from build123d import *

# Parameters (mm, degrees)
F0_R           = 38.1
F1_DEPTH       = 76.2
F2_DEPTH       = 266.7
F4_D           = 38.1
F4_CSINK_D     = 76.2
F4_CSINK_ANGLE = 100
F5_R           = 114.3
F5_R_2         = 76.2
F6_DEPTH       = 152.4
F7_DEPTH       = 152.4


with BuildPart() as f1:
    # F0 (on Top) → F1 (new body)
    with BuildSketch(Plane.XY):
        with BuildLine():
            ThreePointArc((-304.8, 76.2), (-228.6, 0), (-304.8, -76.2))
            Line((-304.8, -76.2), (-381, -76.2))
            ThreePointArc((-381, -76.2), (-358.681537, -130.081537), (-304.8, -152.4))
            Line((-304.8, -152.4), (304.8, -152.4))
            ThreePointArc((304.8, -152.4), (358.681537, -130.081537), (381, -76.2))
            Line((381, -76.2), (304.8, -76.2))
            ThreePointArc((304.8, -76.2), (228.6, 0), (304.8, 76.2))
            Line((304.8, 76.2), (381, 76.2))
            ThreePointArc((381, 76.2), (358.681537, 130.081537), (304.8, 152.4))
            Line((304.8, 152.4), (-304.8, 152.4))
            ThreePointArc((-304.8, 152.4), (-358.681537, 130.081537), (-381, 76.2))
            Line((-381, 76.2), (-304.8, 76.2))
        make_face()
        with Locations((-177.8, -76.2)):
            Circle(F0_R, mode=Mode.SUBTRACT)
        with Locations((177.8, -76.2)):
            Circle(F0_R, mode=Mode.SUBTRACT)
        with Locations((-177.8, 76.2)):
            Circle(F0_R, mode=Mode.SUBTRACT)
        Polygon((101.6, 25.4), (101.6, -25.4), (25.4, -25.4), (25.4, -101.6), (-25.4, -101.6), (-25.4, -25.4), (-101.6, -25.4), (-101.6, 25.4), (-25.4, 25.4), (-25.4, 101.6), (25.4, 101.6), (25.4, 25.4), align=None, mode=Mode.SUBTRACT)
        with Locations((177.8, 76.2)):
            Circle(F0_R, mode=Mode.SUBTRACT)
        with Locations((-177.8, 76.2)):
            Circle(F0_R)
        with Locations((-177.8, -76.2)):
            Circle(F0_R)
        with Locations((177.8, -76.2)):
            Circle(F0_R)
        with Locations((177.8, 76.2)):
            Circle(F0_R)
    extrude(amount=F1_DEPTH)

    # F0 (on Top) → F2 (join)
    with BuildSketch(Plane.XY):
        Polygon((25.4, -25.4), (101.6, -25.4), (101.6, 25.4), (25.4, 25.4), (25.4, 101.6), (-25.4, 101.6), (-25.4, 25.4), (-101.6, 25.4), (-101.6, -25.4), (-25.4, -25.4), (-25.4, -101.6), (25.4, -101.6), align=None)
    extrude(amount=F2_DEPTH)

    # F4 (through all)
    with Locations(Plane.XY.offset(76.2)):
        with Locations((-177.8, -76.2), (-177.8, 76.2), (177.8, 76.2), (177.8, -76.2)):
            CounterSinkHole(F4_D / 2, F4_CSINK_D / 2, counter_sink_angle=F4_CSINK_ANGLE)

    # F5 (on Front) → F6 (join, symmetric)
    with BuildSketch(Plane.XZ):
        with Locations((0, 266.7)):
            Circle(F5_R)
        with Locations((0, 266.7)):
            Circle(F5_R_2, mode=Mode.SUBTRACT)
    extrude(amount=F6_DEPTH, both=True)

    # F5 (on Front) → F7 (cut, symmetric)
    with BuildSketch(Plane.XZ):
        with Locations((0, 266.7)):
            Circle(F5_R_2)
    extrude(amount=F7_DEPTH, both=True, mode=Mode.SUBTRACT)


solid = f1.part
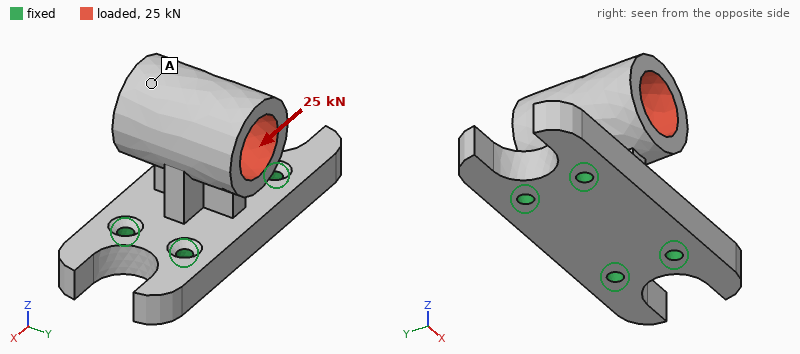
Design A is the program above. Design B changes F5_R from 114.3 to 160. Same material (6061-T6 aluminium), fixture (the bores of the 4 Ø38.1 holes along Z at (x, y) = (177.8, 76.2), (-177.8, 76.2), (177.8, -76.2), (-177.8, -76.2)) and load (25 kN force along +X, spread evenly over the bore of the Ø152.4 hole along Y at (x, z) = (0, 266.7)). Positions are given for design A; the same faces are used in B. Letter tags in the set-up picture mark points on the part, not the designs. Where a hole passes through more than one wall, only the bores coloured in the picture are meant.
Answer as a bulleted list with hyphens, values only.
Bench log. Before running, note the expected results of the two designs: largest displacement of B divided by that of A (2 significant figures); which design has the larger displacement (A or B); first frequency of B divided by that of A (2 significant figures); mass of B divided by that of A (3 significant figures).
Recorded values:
- 0.79
- A
- 0.66
- 1.50
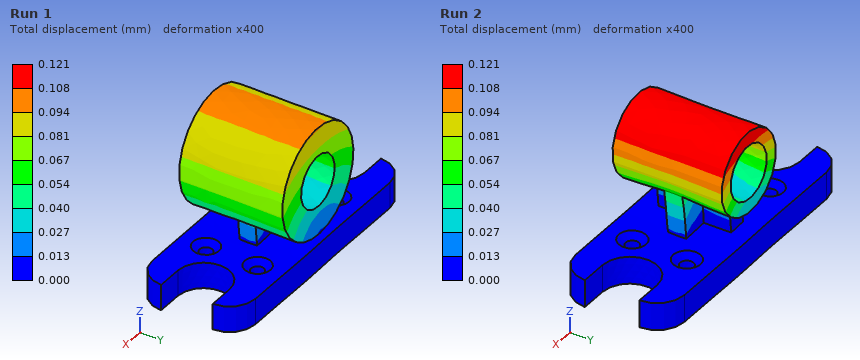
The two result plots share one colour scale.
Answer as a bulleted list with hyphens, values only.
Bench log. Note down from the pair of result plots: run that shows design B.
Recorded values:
- Run 1
